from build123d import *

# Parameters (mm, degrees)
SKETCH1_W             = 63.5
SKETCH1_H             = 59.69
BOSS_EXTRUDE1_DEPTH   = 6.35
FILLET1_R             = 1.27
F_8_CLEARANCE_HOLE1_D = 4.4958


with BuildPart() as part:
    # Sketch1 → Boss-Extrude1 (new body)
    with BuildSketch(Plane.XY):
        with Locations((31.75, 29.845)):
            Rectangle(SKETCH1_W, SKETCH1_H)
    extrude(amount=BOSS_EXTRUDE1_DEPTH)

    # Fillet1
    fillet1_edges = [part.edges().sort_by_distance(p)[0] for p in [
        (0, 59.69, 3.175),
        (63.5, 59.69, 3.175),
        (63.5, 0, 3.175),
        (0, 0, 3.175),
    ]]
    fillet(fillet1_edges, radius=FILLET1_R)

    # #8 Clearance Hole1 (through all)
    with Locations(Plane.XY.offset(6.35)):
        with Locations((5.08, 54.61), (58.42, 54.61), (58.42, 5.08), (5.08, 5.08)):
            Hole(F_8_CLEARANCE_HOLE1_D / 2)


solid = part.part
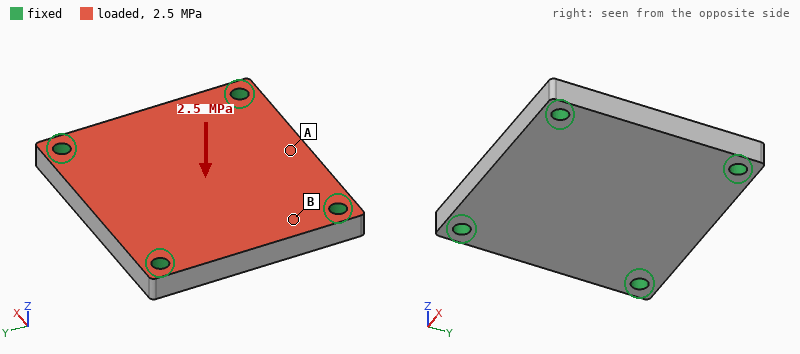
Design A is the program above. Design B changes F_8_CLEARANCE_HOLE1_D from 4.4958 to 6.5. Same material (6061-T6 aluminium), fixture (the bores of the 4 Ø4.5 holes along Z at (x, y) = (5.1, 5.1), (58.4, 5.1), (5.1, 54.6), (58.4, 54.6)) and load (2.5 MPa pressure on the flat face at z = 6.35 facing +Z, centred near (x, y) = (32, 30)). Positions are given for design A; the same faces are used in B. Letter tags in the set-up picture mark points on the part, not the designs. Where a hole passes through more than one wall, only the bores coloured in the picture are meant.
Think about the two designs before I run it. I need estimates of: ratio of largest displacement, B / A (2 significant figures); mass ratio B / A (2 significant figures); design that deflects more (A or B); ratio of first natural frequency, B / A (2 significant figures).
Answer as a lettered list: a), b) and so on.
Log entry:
a) 0.84
b) 0.98
c) A
d) 1.1
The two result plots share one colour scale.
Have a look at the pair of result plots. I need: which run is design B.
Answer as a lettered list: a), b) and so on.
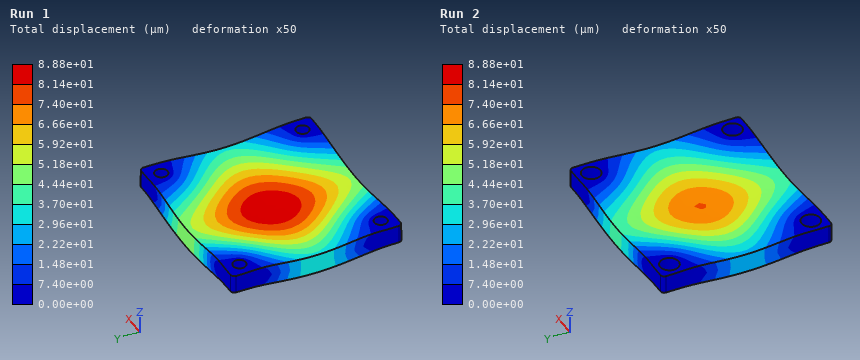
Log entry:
a) Run 2
